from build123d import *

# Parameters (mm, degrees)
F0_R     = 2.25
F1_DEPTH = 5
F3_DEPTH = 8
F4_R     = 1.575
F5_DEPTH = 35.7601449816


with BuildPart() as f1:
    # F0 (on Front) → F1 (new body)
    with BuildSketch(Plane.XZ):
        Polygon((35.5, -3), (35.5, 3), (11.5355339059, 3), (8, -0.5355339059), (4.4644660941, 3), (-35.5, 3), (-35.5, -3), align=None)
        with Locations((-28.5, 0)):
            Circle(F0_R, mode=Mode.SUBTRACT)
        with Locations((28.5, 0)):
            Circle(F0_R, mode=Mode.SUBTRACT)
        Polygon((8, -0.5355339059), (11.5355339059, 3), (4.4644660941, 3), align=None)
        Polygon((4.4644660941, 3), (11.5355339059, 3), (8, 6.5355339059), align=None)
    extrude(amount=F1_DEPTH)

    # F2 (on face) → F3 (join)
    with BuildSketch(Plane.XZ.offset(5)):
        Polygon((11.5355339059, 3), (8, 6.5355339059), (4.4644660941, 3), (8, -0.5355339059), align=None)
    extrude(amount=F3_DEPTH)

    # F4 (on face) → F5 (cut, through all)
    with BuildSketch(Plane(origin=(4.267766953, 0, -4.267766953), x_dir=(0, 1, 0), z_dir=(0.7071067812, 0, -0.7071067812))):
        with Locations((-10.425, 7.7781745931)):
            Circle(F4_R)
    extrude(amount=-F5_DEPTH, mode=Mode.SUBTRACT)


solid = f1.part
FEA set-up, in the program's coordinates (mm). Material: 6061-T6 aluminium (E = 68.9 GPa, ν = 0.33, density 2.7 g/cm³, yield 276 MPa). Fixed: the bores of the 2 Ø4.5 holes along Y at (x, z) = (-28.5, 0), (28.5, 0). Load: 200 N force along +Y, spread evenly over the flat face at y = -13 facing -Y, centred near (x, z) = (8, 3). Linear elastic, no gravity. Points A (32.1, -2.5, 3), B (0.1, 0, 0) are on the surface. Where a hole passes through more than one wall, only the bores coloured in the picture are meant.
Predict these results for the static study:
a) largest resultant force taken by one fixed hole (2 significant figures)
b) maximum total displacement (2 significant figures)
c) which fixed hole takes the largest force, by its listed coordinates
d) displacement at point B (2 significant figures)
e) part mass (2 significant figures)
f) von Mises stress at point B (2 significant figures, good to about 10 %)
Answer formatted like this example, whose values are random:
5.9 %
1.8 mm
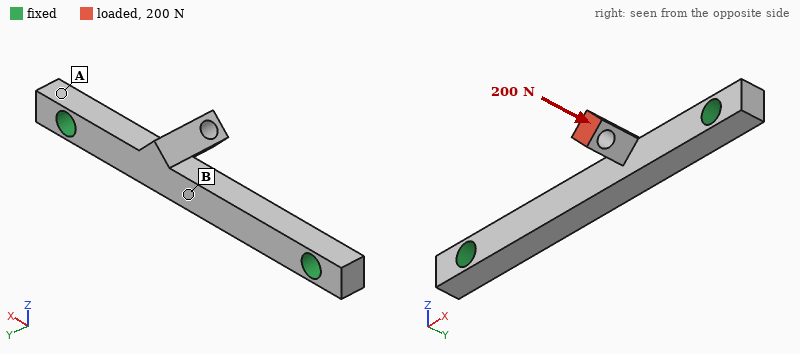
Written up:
140 N
52 µm
(28.5, 0)
31 µm
5.9 g
29 MPa
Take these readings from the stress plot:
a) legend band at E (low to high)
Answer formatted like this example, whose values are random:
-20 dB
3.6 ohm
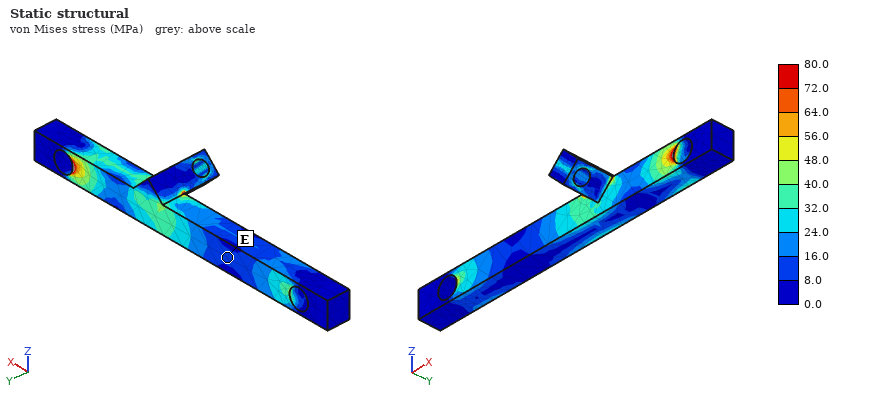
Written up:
8.0 to 16.0 MPa
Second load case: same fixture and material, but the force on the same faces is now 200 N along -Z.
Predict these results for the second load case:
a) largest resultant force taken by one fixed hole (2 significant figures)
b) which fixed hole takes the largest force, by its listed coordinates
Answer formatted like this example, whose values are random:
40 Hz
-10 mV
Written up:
140 N
(28.5, 0)
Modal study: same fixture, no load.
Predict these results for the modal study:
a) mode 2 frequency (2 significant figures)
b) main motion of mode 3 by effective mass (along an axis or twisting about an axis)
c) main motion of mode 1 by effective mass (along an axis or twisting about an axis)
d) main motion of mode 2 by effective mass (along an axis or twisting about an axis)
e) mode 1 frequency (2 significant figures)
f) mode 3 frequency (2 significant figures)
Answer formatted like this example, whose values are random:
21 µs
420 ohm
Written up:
8600 Hz
twisting about X
along Y
along Z
7700 Hz
14 kHz
